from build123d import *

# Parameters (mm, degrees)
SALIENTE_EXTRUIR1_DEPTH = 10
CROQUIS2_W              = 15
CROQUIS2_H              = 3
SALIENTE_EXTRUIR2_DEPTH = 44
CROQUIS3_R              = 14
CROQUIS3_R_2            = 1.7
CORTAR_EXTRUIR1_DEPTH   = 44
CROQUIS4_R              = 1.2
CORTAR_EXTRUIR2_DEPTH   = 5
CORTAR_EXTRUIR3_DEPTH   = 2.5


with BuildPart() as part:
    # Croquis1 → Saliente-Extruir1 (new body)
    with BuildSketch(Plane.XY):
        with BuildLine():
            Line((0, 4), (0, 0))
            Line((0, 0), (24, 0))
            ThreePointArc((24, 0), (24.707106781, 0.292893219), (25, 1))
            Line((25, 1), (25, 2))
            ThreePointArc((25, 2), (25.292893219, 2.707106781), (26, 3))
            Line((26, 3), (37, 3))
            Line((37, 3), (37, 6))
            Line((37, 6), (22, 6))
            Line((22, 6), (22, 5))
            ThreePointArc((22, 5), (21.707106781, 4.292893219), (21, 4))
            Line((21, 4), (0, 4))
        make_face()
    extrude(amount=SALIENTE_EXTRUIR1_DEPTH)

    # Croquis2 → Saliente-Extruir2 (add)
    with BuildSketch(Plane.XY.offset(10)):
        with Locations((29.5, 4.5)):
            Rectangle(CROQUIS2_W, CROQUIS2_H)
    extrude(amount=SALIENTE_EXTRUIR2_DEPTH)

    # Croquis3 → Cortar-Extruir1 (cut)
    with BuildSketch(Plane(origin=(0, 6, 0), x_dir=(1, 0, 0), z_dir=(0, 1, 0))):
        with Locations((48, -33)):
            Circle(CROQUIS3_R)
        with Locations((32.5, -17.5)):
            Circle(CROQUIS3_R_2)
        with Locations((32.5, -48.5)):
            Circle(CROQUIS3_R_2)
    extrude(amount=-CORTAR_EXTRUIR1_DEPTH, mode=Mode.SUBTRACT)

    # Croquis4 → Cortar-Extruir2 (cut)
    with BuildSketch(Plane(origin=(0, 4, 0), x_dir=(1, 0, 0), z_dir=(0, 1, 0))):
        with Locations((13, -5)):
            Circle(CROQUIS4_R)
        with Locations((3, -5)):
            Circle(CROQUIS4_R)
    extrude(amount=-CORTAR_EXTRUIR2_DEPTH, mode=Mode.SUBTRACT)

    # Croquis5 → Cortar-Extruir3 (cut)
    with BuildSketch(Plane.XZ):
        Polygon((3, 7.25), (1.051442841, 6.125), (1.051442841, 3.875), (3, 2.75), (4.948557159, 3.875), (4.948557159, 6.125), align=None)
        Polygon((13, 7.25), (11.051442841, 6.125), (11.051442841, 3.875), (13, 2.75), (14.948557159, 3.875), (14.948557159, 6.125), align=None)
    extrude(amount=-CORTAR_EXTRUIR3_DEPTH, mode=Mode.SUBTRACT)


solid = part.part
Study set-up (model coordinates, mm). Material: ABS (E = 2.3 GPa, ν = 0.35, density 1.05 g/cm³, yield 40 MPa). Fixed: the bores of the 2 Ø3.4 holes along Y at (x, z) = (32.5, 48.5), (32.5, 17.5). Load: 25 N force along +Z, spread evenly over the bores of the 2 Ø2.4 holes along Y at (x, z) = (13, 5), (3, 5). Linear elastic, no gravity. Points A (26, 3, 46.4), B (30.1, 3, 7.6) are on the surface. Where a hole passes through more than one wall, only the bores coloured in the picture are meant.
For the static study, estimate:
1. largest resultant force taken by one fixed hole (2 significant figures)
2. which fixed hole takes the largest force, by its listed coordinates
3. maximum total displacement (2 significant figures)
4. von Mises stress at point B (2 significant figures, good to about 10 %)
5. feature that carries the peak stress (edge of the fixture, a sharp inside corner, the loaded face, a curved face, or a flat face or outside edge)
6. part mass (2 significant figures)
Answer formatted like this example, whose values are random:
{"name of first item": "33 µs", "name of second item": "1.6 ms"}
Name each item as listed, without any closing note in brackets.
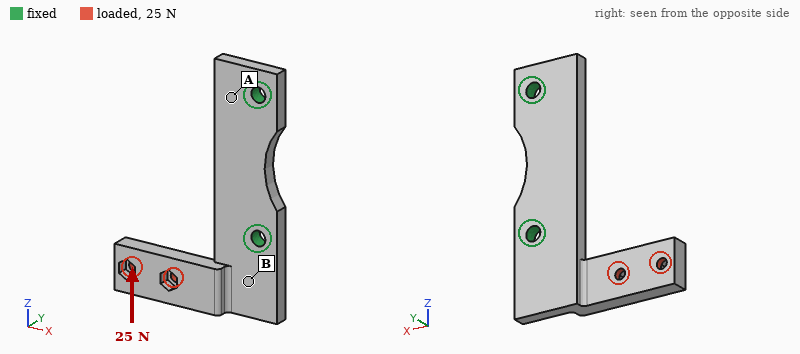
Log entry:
{"largest resultant force taken by one fixed hole": "29 N", "which fixed hole takes the largest force, by its listed coordinates": "(32.5, 48.5)", "maximum total displacement": "0.38 mm", "von Mises stress at point B": "2.4 MPa", "feature that carries the peak stress": "a curved face", "part mass": "3.3 g"}
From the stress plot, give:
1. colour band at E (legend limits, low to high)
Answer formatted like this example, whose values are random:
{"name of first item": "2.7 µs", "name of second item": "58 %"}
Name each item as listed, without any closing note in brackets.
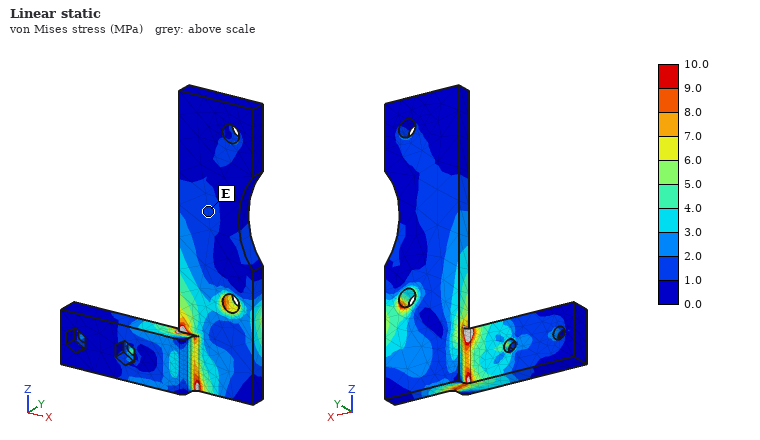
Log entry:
{"colour band at E": "1.0 to 2.0 MPa"}
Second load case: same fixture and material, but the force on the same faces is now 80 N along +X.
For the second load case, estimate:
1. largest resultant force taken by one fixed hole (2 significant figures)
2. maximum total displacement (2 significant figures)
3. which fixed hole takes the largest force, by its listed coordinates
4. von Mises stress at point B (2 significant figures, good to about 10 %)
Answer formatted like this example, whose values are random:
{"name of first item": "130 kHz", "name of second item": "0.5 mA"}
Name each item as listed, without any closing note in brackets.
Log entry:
{"largest resultant force taken by one fixed hole": "110 N", "maximum total displacement": "0.39 mm", "which fixed hole takes the largest force, by its listed coordinates": "(32.5, 17.5)", "von Mises stress at point B": "6.3 MPa"}
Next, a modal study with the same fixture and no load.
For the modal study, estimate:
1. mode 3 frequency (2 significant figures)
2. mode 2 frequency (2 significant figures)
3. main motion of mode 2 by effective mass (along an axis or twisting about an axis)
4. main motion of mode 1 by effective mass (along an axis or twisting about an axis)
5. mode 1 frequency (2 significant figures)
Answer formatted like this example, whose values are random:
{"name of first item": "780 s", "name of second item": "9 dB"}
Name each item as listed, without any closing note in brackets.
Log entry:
{"mode 3 frequency": "2100 Hz", "mode 2 frequency": "1700 Hz", "main motion of mode 2 by effective mass": "along Z", "main motion of mode 1 by effective mass": "along Y", "mode 1 frequency": "640 Hz"}
